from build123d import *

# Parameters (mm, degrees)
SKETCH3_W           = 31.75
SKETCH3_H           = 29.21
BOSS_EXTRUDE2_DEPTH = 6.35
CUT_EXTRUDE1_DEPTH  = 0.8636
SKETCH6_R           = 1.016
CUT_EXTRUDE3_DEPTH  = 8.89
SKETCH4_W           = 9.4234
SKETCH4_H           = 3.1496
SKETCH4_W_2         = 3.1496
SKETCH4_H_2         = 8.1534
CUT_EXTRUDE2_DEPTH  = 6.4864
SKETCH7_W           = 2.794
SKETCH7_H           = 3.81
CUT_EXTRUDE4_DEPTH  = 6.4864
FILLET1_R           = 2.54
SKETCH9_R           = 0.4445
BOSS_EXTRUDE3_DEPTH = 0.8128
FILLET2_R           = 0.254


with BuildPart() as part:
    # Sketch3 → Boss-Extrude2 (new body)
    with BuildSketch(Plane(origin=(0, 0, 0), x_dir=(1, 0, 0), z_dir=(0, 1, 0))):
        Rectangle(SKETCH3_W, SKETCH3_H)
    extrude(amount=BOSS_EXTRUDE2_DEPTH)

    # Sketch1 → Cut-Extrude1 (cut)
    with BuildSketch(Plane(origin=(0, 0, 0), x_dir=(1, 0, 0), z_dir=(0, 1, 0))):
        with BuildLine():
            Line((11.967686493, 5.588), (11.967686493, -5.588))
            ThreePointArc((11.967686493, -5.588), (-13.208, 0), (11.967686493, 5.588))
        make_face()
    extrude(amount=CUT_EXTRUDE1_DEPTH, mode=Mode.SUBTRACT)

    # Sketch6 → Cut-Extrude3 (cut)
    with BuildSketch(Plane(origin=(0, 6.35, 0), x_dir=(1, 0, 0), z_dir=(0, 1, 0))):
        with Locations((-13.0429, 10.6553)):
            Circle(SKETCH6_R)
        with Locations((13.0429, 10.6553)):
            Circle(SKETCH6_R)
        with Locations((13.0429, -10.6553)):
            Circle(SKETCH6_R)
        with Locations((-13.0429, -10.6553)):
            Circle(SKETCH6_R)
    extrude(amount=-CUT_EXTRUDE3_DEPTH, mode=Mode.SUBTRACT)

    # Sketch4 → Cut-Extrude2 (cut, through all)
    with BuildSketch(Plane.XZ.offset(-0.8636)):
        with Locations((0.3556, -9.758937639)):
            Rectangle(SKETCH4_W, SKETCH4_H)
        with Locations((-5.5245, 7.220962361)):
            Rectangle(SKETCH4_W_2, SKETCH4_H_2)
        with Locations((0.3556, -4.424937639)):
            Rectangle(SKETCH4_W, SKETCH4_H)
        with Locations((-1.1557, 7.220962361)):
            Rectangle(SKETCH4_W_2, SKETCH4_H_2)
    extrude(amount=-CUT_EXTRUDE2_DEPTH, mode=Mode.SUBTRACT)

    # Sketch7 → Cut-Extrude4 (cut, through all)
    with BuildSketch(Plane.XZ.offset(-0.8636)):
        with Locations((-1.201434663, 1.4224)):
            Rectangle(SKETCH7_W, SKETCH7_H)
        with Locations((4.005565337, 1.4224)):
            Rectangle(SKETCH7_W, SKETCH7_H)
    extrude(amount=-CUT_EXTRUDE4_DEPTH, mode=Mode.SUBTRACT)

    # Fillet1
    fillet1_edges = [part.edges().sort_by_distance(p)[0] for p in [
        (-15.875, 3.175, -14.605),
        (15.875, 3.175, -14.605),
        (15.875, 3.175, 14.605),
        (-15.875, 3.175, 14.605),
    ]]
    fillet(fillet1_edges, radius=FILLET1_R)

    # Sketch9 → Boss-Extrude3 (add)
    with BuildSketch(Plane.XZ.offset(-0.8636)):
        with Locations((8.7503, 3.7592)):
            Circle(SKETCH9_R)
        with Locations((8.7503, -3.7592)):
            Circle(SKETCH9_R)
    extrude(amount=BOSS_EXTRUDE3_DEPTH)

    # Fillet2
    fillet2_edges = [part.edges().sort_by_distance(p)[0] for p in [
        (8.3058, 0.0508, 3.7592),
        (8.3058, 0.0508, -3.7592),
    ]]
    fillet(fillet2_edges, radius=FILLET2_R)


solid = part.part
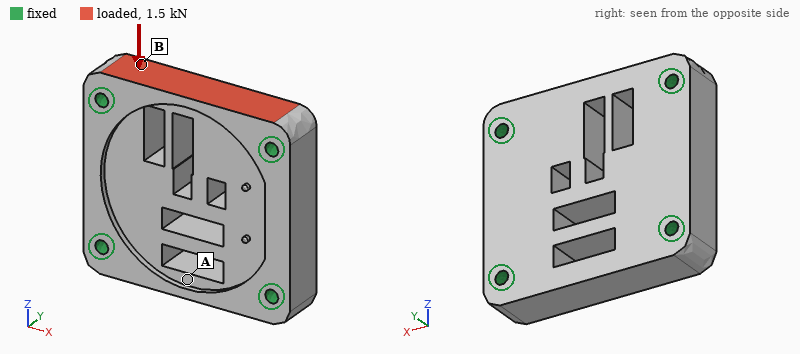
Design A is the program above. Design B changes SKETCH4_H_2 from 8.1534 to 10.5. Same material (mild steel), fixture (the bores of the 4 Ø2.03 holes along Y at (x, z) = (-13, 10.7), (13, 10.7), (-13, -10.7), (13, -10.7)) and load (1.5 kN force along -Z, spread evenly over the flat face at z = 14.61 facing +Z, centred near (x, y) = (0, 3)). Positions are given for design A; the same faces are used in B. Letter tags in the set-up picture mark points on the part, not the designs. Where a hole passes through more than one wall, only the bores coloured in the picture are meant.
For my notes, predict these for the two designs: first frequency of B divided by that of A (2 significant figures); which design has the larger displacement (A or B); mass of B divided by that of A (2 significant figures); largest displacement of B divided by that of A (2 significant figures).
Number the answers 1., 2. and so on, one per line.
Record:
1. 0.99
2. B
3. 0.99
4. 1.2
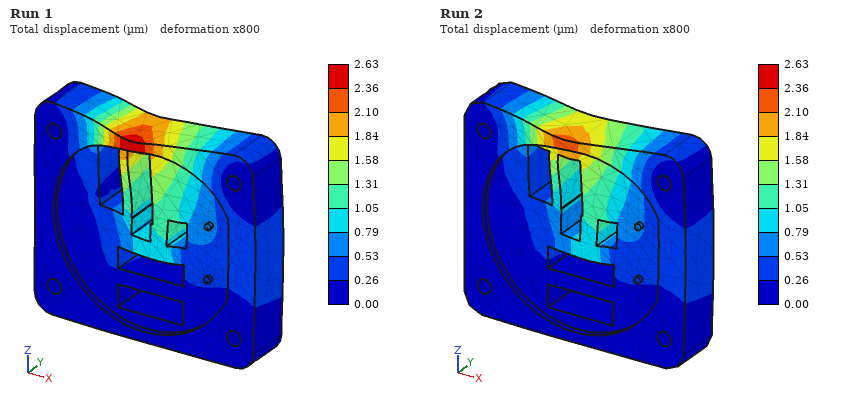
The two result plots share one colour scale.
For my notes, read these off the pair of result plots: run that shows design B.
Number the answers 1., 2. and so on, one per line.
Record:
1. Run 1
